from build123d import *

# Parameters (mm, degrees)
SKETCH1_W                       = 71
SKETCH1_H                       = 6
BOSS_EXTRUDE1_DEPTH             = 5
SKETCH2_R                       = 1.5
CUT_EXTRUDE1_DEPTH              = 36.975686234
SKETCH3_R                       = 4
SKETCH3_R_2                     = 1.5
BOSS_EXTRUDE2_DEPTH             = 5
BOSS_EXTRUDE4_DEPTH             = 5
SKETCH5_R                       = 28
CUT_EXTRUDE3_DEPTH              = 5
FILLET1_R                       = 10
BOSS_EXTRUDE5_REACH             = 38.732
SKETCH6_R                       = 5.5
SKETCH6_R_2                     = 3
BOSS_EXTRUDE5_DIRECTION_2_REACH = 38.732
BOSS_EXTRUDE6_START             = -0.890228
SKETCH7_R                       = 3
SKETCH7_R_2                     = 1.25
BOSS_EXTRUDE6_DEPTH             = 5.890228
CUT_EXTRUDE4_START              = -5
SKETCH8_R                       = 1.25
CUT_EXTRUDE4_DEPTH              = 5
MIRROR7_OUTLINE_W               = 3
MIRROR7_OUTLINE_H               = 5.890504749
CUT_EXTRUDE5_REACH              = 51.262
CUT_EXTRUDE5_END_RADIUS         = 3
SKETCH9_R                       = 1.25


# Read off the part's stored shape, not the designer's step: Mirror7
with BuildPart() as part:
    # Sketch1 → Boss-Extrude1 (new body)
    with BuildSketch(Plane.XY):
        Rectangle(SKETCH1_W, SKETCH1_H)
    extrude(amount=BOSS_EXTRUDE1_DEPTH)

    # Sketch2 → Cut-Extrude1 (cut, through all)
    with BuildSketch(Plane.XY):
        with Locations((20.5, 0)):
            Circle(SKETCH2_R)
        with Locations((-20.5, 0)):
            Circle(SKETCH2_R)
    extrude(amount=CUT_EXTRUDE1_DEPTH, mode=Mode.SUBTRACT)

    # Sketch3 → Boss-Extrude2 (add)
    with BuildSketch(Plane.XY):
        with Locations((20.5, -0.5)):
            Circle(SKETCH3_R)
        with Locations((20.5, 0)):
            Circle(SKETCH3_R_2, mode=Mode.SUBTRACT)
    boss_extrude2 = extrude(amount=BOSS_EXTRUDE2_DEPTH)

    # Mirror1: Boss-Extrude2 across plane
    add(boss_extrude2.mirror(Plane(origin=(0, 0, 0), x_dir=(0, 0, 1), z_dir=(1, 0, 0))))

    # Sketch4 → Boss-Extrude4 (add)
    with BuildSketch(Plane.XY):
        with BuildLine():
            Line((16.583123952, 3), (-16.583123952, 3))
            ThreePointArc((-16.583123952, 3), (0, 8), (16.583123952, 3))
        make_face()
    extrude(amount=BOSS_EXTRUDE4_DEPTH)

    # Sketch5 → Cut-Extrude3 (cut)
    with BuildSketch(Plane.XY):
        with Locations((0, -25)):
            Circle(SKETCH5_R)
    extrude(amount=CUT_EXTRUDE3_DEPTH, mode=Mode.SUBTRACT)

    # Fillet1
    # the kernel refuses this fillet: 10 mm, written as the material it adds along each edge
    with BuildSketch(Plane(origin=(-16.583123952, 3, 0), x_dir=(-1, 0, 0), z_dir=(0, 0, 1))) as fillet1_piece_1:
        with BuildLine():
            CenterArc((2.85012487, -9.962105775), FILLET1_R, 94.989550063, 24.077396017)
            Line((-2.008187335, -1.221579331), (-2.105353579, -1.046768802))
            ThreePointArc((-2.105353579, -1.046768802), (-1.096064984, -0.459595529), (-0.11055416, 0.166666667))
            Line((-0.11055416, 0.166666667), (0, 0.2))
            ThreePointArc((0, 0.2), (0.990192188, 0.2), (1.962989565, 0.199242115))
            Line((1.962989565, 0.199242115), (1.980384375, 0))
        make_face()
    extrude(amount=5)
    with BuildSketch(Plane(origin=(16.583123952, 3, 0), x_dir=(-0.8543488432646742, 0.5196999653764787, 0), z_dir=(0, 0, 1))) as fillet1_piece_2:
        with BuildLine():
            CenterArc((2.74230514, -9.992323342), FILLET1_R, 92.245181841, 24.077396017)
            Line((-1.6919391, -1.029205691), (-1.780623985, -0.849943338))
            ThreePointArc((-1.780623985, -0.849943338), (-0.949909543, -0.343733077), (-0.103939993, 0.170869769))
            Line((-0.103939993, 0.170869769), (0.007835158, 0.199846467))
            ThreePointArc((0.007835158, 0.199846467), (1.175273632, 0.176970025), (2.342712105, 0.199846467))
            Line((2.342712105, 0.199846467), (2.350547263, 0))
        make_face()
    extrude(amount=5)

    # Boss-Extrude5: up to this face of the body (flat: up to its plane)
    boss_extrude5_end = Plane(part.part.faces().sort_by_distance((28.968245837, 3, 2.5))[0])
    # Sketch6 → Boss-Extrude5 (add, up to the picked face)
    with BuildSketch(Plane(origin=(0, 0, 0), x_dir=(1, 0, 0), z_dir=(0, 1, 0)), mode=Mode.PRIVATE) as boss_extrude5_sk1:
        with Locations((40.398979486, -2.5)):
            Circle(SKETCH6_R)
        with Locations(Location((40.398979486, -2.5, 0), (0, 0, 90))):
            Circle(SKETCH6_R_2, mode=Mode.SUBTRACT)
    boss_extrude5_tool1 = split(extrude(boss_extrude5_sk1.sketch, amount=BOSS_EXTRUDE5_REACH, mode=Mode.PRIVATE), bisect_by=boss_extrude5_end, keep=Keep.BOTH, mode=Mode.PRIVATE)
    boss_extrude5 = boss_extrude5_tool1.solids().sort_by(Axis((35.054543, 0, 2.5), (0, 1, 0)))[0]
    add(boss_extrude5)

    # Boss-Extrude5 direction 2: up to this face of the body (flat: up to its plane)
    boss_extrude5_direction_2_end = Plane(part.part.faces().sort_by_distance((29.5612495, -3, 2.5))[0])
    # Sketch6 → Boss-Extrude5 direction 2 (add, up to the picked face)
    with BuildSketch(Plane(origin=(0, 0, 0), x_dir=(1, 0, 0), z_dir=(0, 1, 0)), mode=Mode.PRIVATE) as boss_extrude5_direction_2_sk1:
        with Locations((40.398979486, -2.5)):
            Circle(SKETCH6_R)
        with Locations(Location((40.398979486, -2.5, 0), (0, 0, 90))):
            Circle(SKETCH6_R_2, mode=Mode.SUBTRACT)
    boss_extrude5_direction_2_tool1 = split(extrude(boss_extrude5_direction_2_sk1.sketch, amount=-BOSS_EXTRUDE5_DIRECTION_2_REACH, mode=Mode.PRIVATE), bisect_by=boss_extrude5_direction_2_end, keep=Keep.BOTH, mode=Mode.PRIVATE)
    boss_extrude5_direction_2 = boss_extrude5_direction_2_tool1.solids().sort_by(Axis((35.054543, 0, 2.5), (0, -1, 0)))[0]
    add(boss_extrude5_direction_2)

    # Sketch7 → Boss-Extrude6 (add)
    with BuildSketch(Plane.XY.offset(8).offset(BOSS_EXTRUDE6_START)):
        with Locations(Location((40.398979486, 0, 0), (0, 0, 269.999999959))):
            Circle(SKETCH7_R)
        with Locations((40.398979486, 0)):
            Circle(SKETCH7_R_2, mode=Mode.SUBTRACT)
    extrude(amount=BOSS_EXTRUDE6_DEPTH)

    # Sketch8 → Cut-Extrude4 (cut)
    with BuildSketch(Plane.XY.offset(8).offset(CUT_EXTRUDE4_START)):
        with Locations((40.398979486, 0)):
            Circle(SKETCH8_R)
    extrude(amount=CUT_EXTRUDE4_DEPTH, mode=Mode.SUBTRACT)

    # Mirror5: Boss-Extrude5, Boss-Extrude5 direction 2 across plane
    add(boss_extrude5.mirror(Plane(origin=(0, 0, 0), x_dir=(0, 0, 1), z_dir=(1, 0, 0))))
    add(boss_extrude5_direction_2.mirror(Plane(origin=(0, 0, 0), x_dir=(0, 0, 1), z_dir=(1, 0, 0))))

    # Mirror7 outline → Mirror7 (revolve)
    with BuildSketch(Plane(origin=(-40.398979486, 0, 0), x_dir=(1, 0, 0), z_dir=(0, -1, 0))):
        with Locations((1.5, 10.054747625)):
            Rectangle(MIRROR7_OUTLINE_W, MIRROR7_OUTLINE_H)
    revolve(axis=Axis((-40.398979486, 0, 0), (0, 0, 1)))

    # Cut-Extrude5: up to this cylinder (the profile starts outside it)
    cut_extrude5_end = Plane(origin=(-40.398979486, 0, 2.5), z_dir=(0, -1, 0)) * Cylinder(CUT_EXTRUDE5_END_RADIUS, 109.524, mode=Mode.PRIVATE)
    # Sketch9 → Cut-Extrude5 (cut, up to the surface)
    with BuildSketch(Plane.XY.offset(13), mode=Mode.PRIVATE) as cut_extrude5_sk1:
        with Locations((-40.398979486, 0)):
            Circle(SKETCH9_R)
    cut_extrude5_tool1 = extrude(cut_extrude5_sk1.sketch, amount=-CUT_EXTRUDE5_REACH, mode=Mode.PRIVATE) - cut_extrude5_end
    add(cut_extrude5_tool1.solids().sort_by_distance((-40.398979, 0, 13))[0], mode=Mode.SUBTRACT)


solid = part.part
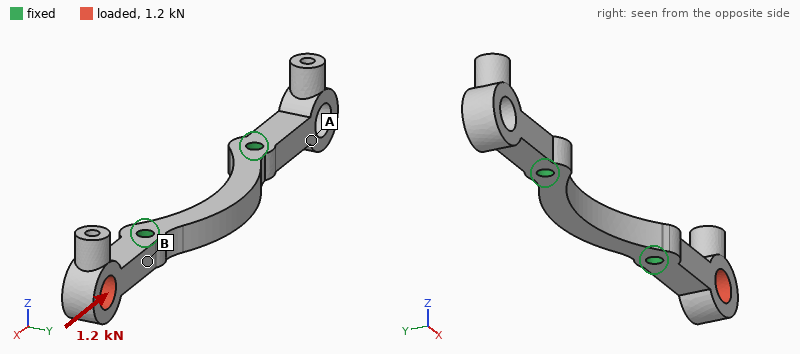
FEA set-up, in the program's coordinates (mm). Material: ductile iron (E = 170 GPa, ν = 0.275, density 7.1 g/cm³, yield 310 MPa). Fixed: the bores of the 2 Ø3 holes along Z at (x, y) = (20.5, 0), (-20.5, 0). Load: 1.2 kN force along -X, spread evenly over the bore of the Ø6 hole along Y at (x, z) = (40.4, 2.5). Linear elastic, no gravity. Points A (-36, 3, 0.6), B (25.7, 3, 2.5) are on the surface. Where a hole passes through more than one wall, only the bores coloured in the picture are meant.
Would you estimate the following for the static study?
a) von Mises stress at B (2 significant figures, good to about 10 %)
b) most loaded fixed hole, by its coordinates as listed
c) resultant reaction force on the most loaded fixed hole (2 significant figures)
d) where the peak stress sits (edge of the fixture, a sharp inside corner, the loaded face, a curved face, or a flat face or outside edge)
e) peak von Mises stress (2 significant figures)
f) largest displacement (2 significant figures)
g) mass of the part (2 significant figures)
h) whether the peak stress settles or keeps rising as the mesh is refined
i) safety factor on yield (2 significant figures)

39 MPa
(20.5, 0)
1.2 kN
the loaded face
180 MPa
9.0 µm
21 g
settles
1.7
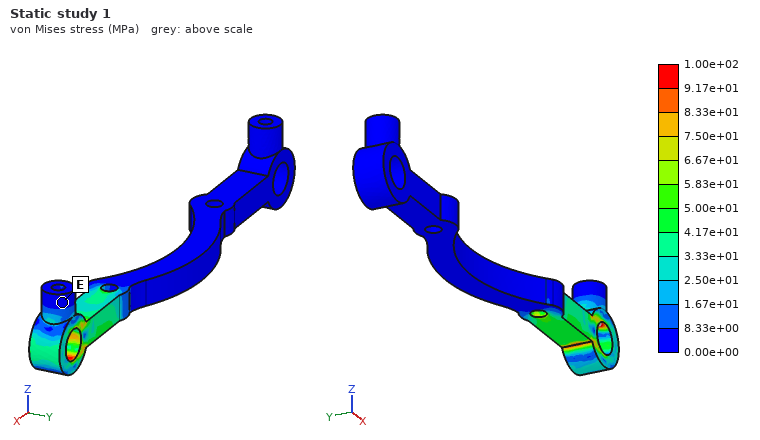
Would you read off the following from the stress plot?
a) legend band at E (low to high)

0.00e+00 to 8.33e+00 MPa
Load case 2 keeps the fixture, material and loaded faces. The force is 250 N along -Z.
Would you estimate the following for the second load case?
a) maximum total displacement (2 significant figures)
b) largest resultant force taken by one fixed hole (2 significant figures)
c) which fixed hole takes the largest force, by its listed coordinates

87 µm
250 N
(20.5, 0)
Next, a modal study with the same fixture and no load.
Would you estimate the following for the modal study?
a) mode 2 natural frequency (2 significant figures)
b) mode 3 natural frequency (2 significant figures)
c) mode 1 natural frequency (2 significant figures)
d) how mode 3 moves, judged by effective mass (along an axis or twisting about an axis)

4900 Hz
5700 Hz
4900 Hz
along Y
